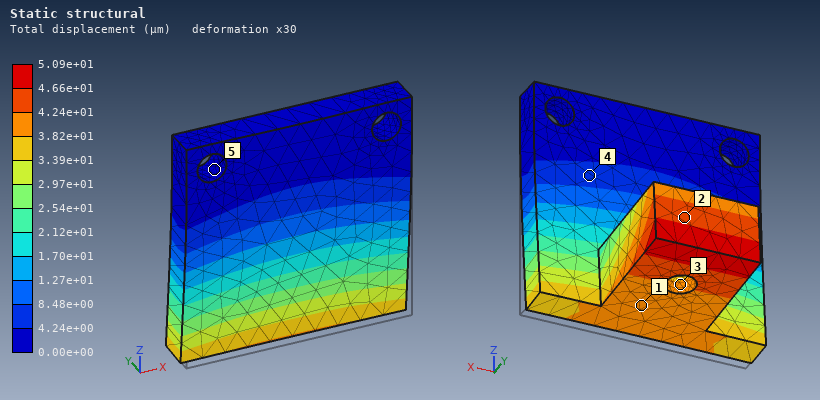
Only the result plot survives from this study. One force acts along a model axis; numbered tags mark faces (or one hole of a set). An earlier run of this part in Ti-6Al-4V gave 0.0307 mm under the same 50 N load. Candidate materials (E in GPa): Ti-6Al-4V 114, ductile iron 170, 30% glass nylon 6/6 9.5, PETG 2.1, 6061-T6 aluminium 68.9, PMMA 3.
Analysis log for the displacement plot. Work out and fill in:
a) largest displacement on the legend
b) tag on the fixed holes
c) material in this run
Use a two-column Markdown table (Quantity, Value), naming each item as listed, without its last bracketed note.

| Quantity | Value |
|---|---|
| largest displacement on the legend | 5.09e+01 µm |
| tag on the fixed holes | 5 |
| material in this run | 6061-T6 aluminium |
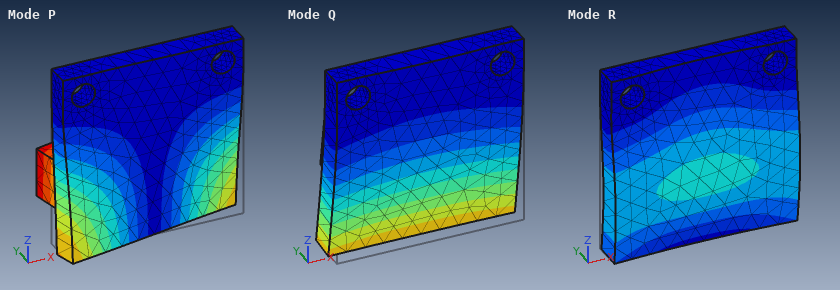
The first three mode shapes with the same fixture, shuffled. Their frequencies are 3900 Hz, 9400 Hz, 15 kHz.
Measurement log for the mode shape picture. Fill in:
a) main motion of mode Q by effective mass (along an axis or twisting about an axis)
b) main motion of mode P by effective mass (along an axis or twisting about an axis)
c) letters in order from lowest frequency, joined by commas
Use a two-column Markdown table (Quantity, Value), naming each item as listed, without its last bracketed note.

| Quantity | Value |
|---|---|
| main motion of mode Q by effective mass | along Y |
| main motion of mode P by effective mass | along X |
| letters in order from lowest frequency, joined by commas | Q, P, R |
